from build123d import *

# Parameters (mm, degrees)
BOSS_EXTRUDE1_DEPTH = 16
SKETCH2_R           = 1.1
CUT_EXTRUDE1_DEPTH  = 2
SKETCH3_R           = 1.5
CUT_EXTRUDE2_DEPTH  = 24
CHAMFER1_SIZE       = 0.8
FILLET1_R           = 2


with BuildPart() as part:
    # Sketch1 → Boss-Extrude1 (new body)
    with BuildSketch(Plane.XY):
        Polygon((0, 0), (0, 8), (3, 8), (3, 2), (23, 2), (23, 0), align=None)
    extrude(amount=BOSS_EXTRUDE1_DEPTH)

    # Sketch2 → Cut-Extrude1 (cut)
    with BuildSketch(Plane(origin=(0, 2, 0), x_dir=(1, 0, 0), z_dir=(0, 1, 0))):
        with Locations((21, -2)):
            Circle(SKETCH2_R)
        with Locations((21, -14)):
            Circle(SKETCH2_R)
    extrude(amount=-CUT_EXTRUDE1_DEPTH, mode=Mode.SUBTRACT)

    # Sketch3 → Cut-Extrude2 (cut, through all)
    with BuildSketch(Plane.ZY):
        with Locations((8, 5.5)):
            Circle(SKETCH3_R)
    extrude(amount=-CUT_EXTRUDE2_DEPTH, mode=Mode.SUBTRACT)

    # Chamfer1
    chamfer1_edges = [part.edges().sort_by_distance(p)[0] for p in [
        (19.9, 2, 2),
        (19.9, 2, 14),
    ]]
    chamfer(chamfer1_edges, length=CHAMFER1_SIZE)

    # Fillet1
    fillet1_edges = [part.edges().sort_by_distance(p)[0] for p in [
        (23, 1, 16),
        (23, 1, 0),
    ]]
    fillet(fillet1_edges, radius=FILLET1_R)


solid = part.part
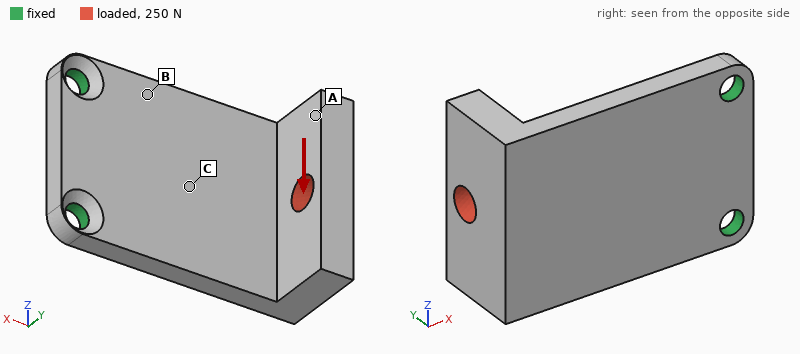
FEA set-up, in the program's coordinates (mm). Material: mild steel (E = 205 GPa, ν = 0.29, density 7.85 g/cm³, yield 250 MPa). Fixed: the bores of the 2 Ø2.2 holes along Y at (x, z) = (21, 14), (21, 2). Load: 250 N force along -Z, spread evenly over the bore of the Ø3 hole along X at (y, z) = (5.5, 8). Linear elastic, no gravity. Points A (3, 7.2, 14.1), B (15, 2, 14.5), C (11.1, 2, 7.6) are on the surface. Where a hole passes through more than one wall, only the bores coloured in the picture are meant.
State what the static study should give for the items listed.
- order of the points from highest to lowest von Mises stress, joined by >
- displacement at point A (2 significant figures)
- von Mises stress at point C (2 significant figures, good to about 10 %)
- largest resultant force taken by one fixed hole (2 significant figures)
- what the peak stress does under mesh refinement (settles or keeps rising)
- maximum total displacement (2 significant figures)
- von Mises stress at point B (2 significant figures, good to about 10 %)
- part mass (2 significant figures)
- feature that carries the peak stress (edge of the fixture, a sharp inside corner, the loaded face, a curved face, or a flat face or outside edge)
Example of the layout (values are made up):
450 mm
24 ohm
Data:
C > B > A
43 µm
100 MPa
420 N
keeps rising
52 µm
76 MPa
7.7 g
edge of the fixture
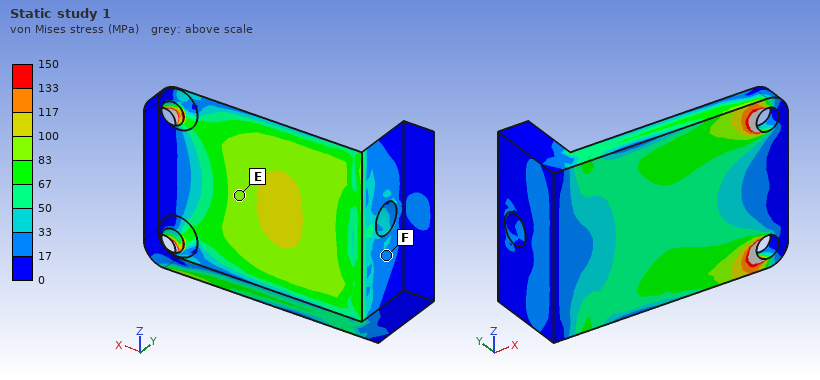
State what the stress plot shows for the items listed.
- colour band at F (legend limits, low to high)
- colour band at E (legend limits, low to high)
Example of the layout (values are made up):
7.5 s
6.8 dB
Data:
17 to 33 MPa
83 to 100 MPa
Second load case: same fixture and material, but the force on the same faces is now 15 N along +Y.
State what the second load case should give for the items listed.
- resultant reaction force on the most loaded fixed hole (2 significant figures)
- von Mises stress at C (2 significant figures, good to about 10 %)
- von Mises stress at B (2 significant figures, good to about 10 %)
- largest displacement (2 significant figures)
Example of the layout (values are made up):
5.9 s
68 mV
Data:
7.7 N
13 MPa
19 MPa
26 µm
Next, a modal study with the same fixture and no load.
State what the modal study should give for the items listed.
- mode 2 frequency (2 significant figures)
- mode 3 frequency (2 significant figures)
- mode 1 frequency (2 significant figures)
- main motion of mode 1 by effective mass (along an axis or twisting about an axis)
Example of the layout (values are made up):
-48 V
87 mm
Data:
6700 Hz
13 kHz
2100 Hz
along Y
